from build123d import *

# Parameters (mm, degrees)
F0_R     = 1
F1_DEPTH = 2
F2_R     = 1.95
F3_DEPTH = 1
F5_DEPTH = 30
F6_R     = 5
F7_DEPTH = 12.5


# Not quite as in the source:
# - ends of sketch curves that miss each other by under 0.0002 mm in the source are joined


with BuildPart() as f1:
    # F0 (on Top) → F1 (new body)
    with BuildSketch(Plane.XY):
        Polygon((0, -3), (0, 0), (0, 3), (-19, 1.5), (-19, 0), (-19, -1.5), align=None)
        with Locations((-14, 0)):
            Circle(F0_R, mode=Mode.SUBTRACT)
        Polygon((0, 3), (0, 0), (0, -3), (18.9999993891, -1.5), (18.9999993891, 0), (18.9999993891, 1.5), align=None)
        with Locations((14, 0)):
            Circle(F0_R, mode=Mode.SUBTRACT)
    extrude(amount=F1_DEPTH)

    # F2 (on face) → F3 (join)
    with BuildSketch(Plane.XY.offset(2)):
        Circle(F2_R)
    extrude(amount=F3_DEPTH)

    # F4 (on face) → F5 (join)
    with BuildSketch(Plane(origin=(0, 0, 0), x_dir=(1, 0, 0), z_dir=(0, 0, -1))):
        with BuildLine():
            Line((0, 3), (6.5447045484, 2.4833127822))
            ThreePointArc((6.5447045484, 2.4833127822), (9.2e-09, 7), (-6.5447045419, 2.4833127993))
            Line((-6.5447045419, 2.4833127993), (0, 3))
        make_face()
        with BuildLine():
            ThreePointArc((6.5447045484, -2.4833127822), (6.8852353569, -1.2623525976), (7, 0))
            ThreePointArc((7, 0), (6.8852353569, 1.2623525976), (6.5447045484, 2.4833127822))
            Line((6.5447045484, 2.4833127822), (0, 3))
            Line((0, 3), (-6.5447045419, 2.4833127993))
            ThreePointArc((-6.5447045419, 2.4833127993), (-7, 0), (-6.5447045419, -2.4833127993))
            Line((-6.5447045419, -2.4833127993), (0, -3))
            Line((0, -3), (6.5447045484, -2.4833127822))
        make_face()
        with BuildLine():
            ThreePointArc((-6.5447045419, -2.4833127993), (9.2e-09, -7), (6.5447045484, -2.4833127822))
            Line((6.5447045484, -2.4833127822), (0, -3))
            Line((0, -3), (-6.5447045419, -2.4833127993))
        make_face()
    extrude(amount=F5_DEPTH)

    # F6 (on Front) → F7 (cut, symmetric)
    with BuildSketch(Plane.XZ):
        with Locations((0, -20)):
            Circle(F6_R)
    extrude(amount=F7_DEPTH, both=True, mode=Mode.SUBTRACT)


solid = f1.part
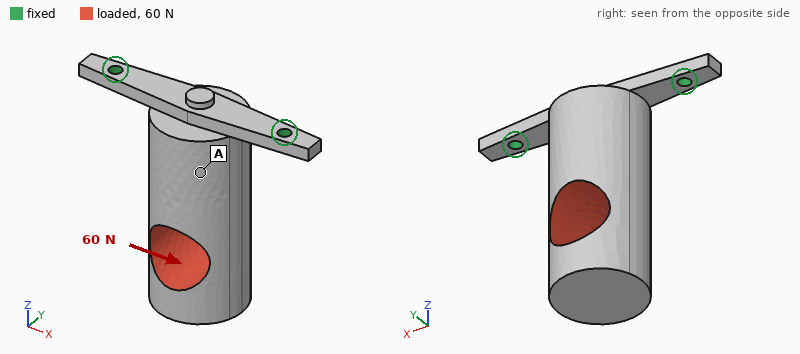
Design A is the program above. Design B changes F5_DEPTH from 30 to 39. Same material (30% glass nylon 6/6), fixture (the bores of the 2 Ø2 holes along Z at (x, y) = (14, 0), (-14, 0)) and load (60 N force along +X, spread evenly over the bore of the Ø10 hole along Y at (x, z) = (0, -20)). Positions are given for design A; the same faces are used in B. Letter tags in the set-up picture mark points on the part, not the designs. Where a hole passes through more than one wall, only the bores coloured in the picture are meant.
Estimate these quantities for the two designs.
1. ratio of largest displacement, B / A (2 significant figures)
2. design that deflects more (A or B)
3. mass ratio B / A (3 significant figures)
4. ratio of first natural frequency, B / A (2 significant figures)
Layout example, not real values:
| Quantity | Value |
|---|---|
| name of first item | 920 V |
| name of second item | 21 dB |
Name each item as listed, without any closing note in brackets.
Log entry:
| Quantity | Value |
|---|---|
| ratio of largest displacement, B / A | 1.3 |
| design that deflects more | B |
| mass ratio B / A | 1.35 |
| ratio of first natural frequency, B / A | 0.62 |
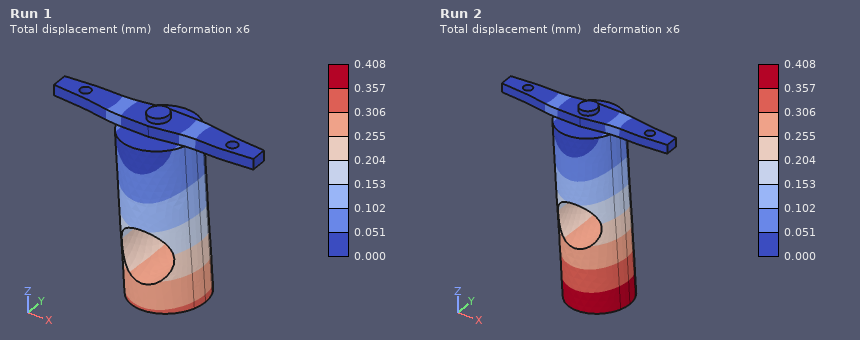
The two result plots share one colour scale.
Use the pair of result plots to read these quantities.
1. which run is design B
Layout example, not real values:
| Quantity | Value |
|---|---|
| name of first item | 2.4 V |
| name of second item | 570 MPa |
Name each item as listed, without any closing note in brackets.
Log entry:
| Quantity | Value |
|---|---|
| which run is design B | Run 2 |
